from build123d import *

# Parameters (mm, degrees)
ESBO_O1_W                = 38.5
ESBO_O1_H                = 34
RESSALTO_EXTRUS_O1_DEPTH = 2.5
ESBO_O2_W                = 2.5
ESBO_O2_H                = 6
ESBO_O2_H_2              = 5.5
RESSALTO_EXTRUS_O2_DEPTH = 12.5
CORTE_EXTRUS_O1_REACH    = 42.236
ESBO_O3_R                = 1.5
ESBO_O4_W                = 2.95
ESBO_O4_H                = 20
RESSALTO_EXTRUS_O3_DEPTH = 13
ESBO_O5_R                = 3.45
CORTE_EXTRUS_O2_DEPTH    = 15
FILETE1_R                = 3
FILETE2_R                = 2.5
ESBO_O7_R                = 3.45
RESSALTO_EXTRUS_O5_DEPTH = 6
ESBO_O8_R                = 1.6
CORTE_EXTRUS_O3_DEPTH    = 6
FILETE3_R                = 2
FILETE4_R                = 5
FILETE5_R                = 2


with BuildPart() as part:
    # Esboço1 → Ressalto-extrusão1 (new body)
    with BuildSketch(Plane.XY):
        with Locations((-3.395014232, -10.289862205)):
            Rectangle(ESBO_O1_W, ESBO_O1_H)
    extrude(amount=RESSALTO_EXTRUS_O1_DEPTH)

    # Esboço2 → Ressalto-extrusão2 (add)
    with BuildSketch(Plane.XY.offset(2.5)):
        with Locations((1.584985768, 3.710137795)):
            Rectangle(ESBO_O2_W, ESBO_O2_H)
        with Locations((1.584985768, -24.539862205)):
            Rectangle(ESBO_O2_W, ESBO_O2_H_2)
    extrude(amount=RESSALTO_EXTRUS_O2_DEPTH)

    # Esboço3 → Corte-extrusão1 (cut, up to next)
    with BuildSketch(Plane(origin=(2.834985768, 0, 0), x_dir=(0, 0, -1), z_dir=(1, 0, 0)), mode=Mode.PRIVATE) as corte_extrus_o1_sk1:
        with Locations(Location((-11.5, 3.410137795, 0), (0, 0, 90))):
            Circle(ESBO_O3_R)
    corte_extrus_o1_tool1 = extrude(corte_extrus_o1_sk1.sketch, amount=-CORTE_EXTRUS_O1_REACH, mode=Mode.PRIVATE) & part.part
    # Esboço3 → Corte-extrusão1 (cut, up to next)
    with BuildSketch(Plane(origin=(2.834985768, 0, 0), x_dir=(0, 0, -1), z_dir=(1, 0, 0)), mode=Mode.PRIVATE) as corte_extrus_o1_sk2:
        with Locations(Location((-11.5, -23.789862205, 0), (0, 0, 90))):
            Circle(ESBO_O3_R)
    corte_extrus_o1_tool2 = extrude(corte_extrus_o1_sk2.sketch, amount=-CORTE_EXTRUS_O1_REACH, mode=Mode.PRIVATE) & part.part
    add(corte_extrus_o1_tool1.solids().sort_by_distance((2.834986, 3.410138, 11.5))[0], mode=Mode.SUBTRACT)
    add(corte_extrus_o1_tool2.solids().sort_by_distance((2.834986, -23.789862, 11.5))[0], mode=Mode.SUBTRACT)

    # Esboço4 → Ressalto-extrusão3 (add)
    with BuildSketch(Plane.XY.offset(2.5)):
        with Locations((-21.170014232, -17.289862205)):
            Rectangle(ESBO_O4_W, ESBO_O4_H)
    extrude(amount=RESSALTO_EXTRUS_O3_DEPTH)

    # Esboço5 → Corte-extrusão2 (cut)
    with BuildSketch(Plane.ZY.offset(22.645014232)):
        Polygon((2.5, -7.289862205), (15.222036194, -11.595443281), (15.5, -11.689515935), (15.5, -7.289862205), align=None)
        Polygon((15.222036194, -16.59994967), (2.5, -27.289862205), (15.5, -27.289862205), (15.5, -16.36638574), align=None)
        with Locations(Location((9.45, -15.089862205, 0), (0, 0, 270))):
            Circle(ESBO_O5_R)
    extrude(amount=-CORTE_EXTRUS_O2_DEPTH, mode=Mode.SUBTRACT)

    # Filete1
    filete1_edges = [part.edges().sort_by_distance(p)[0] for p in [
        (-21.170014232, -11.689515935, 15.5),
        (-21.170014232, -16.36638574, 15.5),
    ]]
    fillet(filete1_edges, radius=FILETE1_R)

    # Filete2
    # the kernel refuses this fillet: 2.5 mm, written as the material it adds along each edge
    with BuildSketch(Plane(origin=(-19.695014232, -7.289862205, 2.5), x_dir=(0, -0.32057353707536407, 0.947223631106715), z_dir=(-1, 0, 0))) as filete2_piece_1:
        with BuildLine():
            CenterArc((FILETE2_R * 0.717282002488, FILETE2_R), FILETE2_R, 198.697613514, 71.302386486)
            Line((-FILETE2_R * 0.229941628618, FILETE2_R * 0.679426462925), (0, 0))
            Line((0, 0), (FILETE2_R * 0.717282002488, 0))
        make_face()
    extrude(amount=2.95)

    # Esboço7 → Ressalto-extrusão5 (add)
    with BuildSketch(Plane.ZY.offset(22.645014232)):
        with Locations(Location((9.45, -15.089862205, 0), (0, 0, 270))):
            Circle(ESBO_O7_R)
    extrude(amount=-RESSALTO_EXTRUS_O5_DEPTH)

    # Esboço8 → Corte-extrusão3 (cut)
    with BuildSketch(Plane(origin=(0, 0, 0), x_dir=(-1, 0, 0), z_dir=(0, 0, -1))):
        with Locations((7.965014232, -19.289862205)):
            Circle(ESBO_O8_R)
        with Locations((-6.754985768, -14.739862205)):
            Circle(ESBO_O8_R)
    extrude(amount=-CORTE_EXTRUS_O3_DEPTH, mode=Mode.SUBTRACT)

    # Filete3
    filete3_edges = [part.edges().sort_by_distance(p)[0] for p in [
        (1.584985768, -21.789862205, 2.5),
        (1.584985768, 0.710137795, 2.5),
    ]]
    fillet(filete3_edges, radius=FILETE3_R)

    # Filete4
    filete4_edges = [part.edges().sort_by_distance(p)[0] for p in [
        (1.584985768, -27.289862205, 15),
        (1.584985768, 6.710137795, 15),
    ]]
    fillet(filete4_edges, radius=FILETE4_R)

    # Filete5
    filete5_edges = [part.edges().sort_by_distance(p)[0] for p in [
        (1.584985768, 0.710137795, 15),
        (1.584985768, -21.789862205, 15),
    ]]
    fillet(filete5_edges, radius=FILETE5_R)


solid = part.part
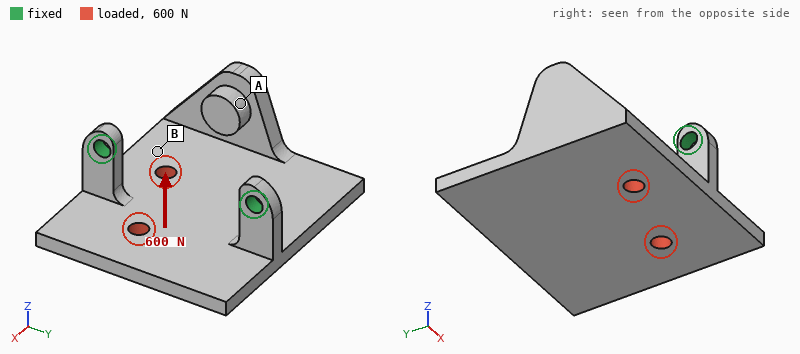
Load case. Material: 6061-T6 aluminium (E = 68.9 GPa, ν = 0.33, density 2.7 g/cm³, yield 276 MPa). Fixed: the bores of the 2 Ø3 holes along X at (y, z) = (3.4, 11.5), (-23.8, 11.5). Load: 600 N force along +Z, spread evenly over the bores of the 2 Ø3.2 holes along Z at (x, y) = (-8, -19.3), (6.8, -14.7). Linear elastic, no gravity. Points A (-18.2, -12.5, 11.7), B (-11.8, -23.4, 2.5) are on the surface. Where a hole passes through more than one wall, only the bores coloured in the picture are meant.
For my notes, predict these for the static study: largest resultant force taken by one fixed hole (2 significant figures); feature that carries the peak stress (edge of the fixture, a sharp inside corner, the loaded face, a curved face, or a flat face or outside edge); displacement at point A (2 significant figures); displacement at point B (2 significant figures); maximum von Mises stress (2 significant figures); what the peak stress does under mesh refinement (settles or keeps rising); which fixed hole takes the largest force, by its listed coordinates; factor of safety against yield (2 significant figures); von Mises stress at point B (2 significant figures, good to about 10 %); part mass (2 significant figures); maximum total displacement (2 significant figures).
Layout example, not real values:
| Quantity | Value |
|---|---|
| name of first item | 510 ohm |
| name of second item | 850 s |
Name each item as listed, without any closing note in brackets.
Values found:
| Quantity | Value |
|---|---|
| largest resultant force taken by one fixed hole | 480 N |
| feature that carries the peak stress | a curved face |
| displacement at point A | 0.33 mm |
| displacement at point B | 0.24 mm |
| maximum von Mises stress | 330 MPa |
| what the peak stress does under mesh refinement | settles |
| which fixed hole takes the largest force, by its listed coordinates | (-23.8, 11.5) |
| factor of safety against yield | 0.85 |
| von Mises stress at point B | 52 MPa |
| part mass | 11 g |
| maximum total displacement | 0.43 mm |
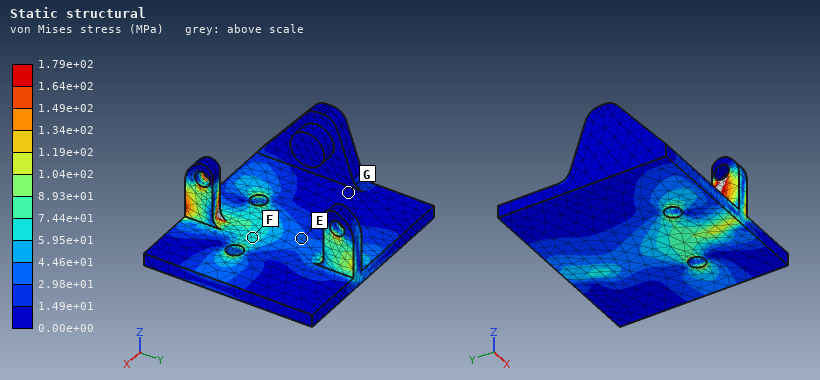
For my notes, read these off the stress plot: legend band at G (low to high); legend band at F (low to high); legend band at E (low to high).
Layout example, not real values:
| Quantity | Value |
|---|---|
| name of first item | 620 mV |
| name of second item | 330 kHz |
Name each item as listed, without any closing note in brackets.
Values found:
| Quantity | Value |
|---|---|
| legend band at G | 0.00e+00 to 1.49e+01 MPa |
| legend band at F | 5.95e+01 to 7.44e+01 MPa |
| legend band at E | 2.98e+01 to 4.46e+01 MPa |
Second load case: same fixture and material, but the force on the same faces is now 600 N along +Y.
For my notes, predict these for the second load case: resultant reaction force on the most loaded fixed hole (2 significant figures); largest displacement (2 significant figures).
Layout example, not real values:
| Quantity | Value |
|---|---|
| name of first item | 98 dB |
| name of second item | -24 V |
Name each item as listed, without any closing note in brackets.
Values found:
| Quantity | Value |
|---|---|
| resultant reaction force on the most loaded fixed hole | 330 N |
| largest displacement | 56 µm |
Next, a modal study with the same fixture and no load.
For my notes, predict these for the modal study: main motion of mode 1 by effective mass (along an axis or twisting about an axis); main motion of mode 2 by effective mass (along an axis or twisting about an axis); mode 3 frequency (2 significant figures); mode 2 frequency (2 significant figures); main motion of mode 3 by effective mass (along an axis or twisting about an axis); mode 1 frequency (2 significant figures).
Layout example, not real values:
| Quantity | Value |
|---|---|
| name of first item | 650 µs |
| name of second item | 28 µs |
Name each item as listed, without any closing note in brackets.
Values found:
| Quantity | Value |
|---|---|
| main motion of mode 1 by effective mass | along Z |
| main motion of mode 2 by effective mass | along Y |
| mode 3 frequency | 4000 Hz |
| mode 2 frequency | 3200 Hz |
| main motion of mode 3 by effective mass | along X |
| mode 1 frequency | 1000 Hz |
